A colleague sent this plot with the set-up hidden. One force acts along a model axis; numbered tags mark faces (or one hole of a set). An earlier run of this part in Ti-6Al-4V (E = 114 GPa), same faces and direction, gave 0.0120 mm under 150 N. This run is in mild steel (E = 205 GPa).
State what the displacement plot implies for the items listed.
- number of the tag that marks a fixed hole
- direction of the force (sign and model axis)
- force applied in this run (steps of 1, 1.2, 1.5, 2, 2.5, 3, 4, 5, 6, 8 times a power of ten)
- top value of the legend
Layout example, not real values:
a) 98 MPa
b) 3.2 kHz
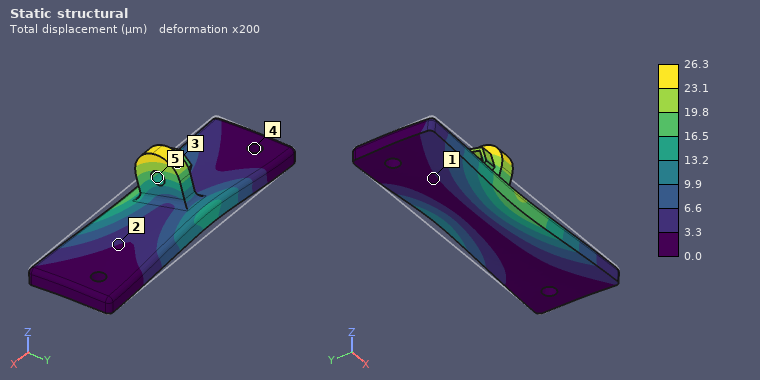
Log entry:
a) 4
b) -Y
c) 600 N
d) 26.3 µm
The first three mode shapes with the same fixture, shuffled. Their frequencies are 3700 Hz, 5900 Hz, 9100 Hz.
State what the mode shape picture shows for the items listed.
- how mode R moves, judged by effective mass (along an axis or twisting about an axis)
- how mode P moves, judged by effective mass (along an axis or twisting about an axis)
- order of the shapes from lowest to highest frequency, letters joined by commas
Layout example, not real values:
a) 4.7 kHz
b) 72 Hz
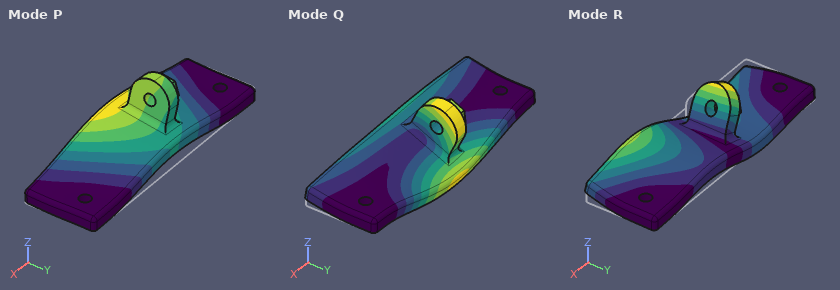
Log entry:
a) twisting about Y
b) along Z
c) P, Q, R
